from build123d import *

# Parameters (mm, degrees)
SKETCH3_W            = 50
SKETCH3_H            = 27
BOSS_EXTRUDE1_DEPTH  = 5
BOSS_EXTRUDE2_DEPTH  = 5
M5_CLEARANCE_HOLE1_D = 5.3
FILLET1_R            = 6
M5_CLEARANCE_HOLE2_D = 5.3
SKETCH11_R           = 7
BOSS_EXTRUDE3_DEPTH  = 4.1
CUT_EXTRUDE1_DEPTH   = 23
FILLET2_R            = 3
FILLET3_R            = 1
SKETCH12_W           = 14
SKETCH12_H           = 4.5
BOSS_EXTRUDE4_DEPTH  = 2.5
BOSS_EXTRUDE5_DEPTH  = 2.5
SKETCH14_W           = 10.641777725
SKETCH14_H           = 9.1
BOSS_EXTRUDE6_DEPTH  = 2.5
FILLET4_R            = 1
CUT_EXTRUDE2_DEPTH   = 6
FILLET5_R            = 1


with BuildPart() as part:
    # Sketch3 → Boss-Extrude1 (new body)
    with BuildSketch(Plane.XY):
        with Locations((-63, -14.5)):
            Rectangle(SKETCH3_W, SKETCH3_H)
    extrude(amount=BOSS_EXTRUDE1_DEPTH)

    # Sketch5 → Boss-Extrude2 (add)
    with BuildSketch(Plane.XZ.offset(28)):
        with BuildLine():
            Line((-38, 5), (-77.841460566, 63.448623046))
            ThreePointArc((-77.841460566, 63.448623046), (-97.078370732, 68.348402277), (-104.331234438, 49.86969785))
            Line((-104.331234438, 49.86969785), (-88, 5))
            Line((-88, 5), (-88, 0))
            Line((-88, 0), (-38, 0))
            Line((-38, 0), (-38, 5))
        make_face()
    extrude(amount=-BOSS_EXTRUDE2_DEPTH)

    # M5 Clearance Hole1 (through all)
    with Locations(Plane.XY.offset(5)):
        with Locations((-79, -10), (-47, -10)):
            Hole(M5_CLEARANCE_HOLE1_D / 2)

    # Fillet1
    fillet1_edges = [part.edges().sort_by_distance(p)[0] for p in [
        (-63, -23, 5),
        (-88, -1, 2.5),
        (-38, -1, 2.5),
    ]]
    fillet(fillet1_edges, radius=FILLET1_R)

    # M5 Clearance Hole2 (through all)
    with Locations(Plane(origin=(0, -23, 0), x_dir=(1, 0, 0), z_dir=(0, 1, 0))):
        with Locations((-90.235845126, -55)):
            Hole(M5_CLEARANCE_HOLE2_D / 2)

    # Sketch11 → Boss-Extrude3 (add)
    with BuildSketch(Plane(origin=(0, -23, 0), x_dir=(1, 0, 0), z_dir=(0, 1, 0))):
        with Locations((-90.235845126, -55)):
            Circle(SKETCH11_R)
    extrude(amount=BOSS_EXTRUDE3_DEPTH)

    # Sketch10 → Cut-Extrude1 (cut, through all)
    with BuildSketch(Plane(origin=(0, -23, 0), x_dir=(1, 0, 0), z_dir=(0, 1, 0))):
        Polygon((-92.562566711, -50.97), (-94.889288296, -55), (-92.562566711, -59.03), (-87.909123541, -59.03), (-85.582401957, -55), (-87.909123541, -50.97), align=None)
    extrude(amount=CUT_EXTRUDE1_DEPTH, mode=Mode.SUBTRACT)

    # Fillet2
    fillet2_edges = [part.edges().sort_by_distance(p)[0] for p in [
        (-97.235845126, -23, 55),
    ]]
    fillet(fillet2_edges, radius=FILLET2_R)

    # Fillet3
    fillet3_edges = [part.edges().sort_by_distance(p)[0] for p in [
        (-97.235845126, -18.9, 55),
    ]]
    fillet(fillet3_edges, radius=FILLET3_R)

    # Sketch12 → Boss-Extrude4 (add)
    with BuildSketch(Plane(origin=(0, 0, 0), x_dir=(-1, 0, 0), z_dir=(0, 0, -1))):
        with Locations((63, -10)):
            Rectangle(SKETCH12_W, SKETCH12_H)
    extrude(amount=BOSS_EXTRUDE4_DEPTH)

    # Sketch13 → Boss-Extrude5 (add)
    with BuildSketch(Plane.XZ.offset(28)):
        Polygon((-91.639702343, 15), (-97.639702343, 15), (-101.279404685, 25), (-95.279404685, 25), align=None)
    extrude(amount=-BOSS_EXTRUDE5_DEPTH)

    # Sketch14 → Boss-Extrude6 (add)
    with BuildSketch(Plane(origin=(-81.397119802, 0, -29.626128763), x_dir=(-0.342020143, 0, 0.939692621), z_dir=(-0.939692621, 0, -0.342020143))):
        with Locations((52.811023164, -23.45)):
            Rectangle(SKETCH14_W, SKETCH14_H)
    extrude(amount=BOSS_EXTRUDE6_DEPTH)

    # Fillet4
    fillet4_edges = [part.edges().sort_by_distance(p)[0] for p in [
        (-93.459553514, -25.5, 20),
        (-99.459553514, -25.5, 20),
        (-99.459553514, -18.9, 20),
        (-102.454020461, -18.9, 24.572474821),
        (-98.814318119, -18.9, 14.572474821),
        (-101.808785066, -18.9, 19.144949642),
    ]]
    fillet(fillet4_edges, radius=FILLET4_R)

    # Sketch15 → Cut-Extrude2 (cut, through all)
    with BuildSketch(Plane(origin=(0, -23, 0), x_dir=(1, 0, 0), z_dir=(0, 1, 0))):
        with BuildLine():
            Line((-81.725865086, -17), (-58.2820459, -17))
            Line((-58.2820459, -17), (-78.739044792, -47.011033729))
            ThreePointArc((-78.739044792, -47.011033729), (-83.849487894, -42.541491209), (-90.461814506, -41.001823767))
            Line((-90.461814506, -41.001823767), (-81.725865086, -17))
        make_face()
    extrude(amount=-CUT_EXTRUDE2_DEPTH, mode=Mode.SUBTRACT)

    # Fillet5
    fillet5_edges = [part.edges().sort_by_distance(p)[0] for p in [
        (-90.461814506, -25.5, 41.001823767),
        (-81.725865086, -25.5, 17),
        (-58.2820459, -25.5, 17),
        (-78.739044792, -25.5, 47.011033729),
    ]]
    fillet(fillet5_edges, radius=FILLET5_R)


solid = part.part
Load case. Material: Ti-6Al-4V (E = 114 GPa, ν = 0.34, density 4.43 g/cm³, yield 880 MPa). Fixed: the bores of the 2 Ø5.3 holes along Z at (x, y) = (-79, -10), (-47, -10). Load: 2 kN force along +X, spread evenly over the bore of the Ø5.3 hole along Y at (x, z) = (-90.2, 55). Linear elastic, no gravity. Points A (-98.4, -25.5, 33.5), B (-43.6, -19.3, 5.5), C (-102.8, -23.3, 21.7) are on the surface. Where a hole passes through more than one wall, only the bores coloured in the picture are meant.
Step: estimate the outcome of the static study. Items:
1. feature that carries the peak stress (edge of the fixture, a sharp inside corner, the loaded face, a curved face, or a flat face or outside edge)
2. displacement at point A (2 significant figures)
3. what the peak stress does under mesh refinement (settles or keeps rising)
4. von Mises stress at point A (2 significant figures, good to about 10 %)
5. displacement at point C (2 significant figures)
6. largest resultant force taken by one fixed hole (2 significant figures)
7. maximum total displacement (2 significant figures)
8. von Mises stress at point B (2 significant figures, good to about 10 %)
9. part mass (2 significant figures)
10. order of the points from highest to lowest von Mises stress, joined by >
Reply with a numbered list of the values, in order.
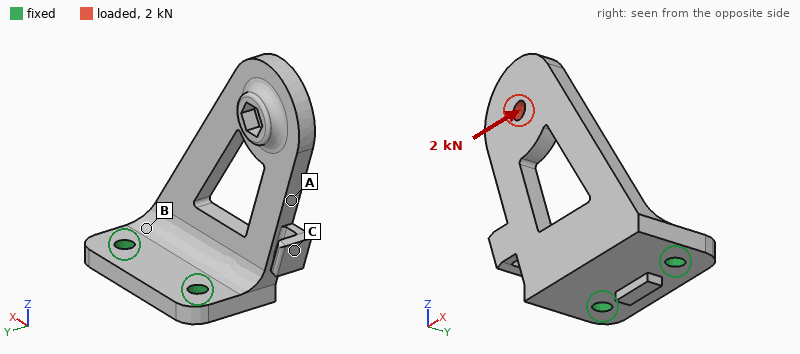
1. edge of the fixture
2. 0.28 mm
3. keeps rising
4. 61 MPa
5. 0.25 mm
6. 3.2 kN
7. 0.42 mm
8. 110 MPa
9. 78 g
10. B > A > C
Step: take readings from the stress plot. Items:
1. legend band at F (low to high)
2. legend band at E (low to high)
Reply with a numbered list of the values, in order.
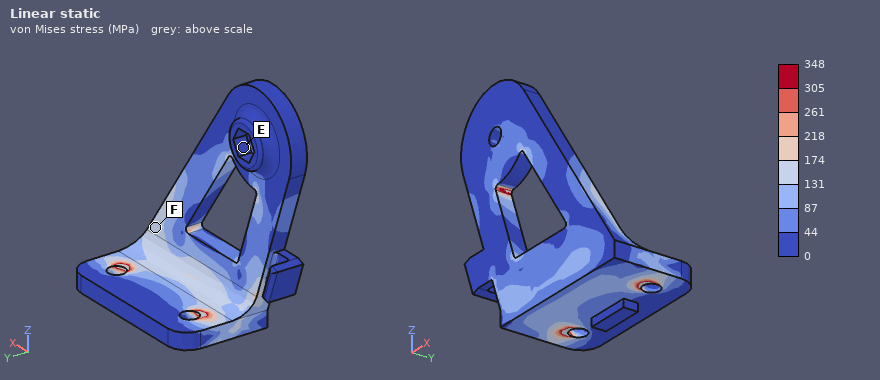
1. 131 to 174 MPa
2. 0 to 44 MPa
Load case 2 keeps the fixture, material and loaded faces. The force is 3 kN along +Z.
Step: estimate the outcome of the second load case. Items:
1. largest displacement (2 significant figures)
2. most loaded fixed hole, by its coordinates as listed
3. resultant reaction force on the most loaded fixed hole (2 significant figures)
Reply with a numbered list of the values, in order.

1. 0.60 mm
2. (-79, -10)
3. 3.8 kN
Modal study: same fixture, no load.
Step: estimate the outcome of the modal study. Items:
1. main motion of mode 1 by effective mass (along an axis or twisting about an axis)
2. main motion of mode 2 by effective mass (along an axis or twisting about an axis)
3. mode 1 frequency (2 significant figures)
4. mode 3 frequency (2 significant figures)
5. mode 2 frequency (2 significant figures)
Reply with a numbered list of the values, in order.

1. along Y
2. along X
3. 730 Hz
4. 3300 Hz
5. 2300 Hz
